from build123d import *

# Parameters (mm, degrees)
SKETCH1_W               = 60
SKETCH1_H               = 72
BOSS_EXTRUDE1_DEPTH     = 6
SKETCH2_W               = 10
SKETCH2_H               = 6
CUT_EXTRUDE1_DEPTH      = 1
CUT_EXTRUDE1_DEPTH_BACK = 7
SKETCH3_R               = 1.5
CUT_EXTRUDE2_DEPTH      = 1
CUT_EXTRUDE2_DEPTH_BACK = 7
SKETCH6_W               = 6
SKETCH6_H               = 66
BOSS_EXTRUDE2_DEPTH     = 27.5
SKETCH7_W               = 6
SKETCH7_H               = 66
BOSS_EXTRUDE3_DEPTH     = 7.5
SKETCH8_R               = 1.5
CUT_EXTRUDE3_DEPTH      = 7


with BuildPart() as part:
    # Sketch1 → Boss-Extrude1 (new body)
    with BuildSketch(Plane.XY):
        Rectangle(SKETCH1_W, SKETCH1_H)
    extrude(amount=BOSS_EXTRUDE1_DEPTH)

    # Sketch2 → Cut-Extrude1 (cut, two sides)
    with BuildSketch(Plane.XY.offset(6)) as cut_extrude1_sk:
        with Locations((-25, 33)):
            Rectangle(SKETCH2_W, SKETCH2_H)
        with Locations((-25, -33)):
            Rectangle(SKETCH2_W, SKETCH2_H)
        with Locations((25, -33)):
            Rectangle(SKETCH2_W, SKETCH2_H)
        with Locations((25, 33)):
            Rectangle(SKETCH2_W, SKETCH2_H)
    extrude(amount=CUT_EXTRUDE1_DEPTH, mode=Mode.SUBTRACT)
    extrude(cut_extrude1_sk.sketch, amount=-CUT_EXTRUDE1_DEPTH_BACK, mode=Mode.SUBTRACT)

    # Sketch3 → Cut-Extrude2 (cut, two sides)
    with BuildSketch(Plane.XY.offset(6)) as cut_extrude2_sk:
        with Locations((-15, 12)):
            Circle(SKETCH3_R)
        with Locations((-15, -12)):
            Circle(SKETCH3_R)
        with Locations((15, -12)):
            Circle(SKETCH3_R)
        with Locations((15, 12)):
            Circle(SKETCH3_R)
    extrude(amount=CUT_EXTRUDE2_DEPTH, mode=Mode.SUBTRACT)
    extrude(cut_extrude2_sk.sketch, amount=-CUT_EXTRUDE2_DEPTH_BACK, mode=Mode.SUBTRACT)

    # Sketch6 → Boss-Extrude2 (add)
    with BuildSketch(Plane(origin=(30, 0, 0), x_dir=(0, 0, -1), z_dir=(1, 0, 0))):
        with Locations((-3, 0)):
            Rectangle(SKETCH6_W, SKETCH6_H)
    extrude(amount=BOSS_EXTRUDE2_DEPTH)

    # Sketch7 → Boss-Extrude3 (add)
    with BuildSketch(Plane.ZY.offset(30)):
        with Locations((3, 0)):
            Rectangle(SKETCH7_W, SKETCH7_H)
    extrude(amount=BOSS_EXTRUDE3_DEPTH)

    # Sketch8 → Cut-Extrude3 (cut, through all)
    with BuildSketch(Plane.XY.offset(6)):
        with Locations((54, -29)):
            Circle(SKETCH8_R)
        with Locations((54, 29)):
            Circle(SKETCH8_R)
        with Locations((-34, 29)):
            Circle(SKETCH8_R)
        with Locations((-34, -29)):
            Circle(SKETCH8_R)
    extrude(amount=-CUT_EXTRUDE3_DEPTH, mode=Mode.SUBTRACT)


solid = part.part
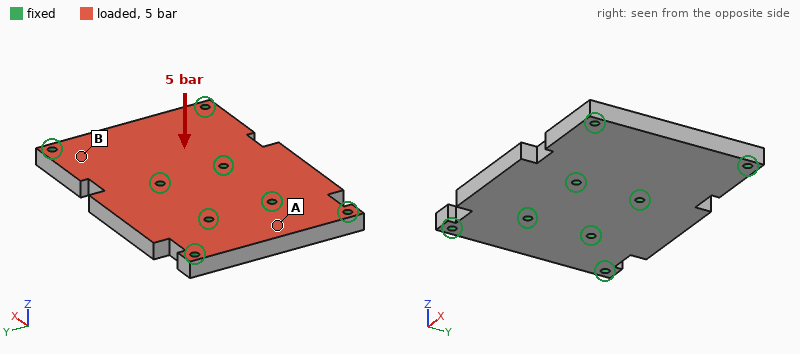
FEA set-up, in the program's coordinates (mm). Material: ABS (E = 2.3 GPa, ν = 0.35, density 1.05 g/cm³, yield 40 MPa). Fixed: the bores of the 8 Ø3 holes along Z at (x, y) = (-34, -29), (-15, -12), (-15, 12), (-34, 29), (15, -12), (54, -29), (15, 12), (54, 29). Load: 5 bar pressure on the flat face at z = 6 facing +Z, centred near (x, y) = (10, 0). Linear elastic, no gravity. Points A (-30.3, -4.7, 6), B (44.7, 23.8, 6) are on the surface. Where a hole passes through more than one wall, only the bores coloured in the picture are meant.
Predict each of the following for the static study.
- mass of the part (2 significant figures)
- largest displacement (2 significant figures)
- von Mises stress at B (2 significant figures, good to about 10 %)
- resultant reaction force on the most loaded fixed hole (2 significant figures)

40 g
0.47 mm
7.7 MPa
640 N
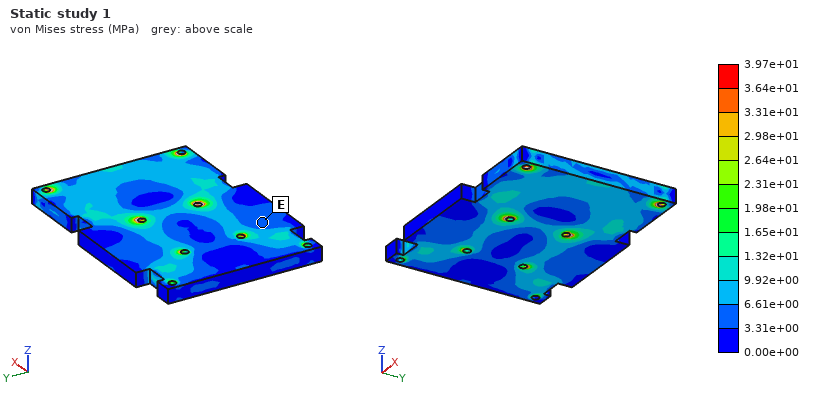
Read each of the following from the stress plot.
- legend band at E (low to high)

3.31e+00 to 6.61e+00 MPa
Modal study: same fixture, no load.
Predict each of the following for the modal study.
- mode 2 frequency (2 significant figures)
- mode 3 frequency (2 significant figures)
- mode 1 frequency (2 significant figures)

2600 Hz
2700 Hz
2400 Hz
